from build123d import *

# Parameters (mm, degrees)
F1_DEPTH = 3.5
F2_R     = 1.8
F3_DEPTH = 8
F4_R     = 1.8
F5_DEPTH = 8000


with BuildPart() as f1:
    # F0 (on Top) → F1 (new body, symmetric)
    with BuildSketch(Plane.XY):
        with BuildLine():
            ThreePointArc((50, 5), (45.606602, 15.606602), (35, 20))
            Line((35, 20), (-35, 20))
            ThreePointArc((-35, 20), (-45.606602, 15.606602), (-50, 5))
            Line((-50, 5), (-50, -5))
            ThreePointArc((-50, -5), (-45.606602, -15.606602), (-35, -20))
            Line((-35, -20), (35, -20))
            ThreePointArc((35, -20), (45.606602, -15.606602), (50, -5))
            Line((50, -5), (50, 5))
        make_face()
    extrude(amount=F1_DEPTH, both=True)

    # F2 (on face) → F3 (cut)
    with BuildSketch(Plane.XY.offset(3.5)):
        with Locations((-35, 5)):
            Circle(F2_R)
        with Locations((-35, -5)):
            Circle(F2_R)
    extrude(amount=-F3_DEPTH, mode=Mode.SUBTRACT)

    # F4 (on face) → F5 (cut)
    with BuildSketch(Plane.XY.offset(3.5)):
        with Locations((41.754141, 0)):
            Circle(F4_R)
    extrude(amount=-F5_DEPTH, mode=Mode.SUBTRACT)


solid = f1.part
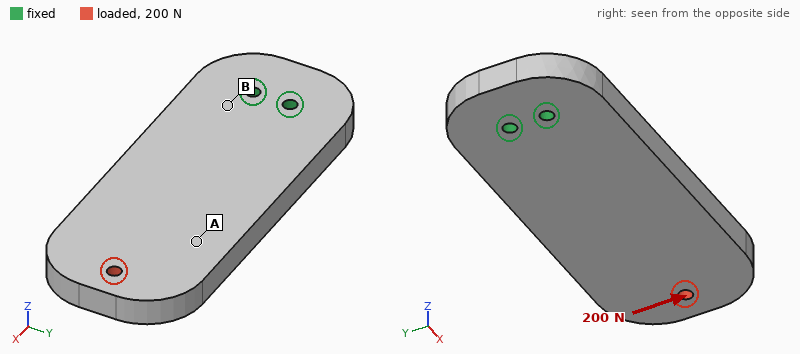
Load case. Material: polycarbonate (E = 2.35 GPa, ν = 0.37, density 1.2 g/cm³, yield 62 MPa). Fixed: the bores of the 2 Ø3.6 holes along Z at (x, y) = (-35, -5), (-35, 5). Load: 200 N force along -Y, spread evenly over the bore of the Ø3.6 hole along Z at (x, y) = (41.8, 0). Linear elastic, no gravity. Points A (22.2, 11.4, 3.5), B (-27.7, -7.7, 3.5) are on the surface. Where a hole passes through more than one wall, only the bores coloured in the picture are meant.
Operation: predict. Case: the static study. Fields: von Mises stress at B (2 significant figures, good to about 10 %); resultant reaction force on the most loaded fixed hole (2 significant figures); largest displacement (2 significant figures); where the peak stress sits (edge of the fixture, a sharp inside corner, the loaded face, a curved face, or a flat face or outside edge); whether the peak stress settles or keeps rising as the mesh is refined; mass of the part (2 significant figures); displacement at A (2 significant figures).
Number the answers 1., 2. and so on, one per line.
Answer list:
1. 7.7 MPa
2. 1.2 kN
3. 1.1 mm
4. edge of the fixture
5. keeps rising
6. 32 g
7. 0.68 mm
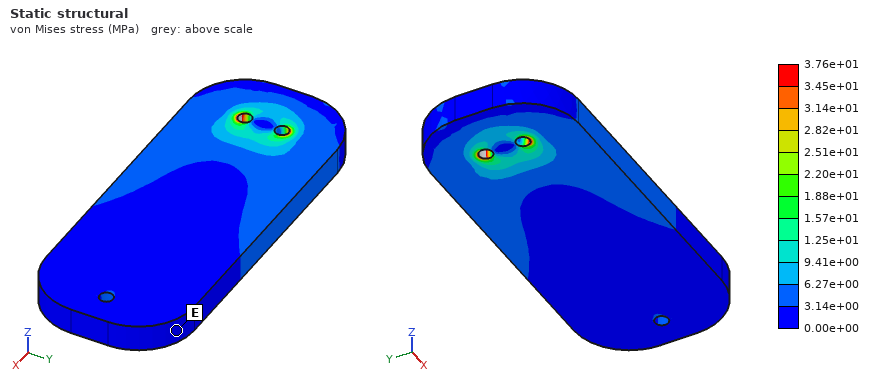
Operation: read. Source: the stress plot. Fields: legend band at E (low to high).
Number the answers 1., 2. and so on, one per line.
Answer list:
1. 0.00e+00 to 3.14e+00 MPa
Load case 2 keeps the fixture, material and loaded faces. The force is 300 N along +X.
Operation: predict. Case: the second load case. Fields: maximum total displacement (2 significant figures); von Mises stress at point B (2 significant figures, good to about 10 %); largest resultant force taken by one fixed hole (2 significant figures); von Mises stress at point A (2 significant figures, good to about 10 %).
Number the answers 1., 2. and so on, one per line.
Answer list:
1. 54 µm
2. 1.5 MPa
3. 150 N
4. 1.1 MPa
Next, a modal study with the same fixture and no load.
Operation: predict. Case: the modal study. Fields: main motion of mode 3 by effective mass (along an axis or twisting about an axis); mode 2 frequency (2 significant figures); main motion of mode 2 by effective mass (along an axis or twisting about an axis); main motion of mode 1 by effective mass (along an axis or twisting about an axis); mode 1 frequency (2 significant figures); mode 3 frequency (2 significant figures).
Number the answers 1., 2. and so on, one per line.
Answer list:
1. twisting about X
2. 720 Hz
3. along Y
4. along Z
5. 230 Hz
6. 910 Hz
